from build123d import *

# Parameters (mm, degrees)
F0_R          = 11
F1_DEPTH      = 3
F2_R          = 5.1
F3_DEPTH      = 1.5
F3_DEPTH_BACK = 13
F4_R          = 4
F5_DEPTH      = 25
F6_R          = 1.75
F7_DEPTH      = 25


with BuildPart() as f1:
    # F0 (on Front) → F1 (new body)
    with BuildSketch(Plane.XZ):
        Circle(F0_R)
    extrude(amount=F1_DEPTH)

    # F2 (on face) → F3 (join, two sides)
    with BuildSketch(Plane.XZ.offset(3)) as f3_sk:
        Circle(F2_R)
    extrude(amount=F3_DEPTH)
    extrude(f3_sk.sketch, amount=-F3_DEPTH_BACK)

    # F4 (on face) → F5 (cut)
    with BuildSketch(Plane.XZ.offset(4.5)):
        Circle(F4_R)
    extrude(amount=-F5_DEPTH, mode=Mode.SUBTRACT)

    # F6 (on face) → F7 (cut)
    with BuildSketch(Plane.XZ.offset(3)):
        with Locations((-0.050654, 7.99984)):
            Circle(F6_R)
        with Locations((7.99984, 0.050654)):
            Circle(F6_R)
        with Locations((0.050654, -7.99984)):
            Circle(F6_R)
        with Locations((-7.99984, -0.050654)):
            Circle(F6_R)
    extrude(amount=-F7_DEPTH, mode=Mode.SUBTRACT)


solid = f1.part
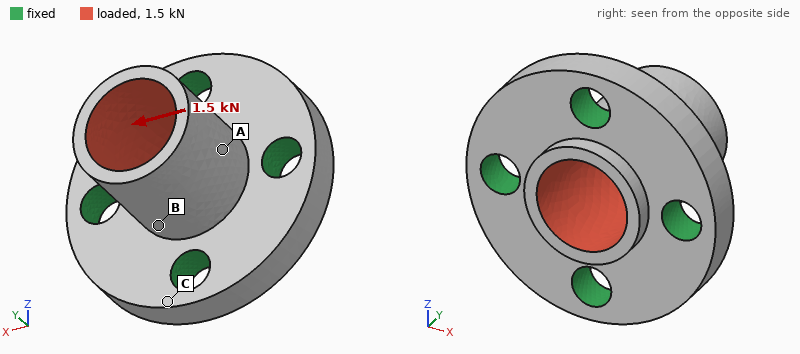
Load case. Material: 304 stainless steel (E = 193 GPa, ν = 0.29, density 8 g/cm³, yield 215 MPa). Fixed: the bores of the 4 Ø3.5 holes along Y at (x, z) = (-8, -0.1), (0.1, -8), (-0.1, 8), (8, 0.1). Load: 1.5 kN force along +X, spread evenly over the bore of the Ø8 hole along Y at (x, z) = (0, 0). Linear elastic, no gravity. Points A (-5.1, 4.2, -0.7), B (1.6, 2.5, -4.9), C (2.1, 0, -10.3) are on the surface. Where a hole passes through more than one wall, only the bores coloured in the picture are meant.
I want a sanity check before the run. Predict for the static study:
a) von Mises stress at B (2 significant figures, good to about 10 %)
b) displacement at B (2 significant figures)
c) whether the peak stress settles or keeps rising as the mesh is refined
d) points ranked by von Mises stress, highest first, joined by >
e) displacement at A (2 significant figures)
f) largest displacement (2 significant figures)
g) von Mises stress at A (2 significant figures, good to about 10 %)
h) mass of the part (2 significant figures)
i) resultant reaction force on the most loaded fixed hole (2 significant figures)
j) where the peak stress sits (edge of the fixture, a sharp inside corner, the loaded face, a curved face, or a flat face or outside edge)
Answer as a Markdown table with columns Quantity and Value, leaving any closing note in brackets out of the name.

| Quantity | Value |
|---|---|
| von Mises stress at B | 62 MPa |
| displacement at B | 3.2 µm |
| whether the peak stress settles or keeps rising as the mesh is refined | keeps rising |
| points ranked by von Mises stress, highest first, joined by > | B > A > C |
| displacement at A | 5.8 µm |
| largest displacement | 10.0 µm |
| von Mises stress at A | 25 MPa |
| mass of the part | 9.9 g |
| resultant reaction force on the most loaded fixed hole | 630 N |
| where the peak stress sits | a sharp inside corner |
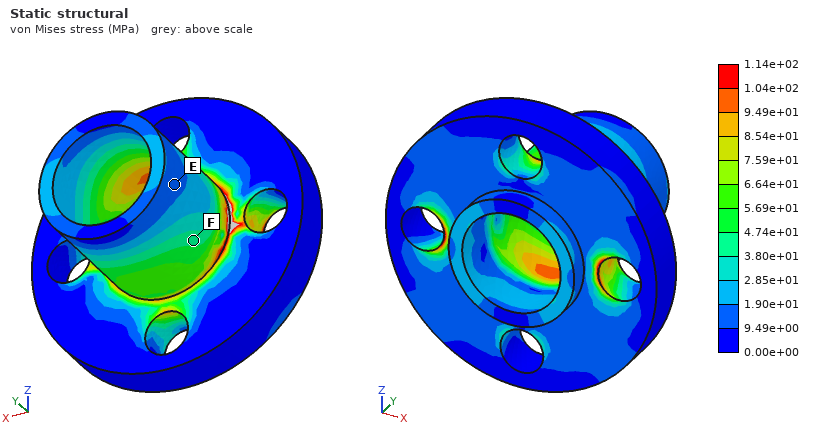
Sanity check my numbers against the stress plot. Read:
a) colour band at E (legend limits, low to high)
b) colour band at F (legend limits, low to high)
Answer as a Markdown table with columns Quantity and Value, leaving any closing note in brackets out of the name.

| Quantity | Value |
|---|---|
| colour band at E | 9.49e+00 to 1.90e+01 MPa |
| colour band at F | 3.80e+01 to 4.74e+01 MPa |
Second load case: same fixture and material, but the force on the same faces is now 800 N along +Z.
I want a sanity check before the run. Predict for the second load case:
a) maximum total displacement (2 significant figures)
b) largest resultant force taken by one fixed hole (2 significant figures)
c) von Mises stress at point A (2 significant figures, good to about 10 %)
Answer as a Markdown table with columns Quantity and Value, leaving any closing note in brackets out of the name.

| Quantity | Value |
|---|---|
| maximum total displacement | 5.3 µm |
| largest resultant force taken by one fixed hole | 340 N |
| von Mises stress at point A | 31 MPa |
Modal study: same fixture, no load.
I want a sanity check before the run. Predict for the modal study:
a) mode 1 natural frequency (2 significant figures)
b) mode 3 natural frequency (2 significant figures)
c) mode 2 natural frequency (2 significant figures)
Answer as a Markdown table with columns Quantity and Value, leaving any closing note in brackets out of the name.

| Quantity | Value |
|---|---|
| mode 1 natural frequency | 38 kHz |
| mode 3 natural frequency | 40 kHz |
| mode 2 natural frequency | 38 kHz |
